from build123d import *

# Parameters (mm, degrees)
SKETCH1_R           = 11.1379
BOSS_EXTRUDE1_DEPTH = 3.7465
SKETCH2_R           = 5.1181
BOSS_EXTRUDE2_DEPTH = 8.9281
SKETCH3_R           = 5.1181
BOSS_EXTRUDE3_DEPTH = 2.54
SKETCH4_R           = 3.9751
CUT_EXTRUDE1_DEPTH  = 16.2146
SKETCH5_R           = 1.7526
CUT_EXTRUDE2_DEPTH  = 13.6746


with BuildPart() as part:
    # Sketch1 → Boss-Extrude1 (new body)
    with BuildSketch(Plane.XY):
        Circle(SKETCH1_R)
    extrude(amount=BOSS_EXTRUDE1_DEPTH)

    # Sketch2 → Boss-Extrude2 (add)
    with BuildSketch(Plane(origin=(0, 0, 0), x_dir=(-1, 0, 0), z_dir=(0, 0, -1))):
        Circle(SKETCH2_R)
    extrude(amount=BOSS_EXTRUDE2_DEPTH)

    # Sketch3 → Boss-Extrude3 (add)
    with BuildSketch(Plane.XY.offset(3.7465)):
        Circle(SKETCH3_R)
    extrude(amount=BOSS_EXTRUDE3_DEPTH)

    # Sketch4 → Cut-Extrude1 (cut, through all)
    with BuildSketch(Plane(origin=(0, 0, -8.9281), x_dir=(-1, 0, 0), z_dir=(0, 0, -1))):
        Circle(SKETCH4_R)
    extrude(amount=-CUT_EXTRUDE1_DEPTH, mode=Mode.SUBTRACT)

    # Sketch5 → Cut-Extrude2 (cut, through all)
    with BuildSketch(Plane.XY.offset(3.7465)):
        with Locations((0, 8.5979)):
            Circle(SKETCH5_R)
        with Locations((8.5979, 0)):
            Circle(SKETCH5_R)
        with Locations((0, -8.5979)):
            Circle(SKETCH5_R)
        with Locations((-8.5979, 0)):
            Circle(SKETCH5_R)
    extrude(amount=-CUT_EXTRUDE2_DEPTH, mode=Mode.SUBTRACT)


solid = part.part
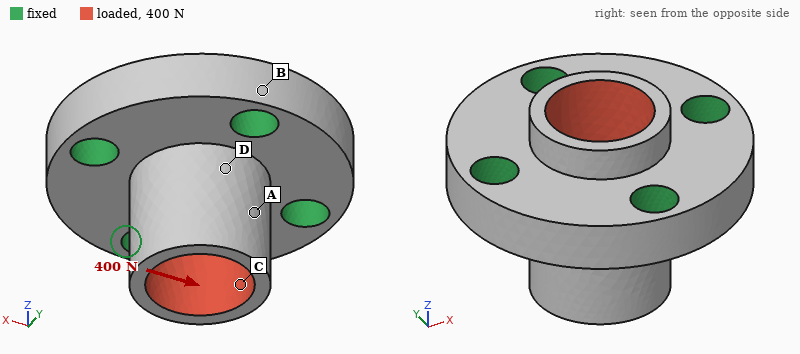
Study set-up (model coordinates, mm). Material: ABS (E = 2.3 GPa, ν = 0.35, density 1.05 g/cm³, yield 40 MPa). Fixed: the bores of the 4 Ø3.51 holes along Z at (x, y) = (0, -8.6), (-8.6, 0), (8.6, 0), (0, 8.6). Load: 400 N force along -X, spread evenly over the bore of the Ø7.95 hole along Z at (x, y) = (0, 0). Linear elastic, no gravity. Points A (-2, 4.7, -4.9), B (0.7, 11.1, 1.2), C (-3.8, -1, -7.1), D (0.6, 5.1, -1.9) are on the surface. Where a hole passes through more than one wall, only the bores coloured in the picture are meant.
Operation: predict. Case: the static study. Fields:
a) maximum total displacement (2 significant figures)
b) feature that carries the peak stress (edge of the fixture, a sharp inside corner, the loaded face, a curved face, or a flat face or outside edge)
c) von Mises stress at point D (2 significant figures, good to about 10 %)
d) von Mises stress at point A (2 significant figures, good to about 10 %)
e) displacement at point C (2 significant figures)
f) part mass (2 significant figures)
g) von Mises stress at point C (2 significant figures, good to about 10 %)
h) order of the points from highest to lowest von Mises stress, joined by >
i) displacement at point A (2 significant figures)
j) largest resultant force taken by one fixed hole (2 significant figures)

0.16 mm
a curved face
14 MPa
9.8 MPa
0.13 mm
1.6 g
5.3 MPa
D > A > C > B
0.095 mm
150 N
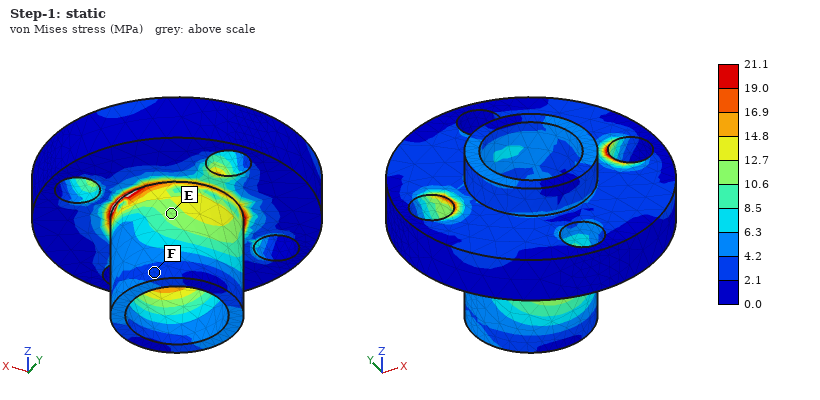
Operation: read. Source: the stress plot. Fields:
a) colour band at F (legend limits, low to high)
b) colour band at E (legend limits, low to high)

2.1 to 4.2 MPa
10.6 to 12.7 MPa
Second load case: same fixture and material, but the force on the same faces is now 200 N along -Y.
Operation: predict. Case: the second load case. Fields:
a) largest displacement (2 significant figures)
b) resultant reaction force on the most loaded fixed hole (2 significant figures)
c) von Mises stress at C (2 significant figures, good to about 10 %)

78 µm
74 N
3.1 MPa
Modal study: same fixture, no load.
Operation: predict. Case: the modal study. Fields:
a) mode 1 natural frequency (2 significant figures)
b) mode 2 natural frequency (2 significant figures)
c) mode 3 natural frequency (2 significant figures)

13 kHz
13 kHz
13 kHz
